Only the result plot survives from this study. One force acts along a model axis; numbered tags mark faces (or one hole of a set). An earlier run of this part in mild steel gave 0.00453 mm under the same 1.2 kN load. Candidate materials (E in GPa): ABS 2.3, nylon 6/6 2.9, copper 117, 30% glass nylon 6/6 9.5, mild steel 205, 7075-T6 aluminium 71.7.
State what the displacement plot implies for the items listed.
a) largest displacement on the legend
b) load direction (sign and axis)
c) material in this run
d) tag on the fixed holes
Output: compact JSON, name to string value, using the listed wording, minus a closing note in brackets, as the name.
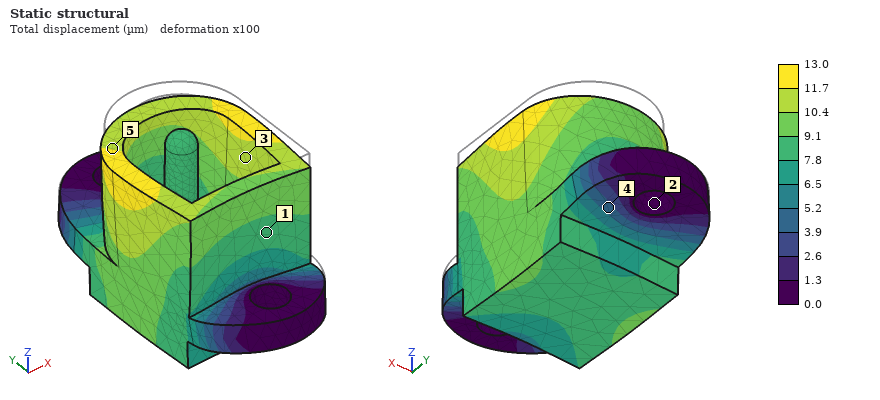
{"largest displacement on the legend": "13.0 µm", "load direction": "-Z", "material in this run": "7075-T6 aluminium", "tag on the fixed holes": "2"}
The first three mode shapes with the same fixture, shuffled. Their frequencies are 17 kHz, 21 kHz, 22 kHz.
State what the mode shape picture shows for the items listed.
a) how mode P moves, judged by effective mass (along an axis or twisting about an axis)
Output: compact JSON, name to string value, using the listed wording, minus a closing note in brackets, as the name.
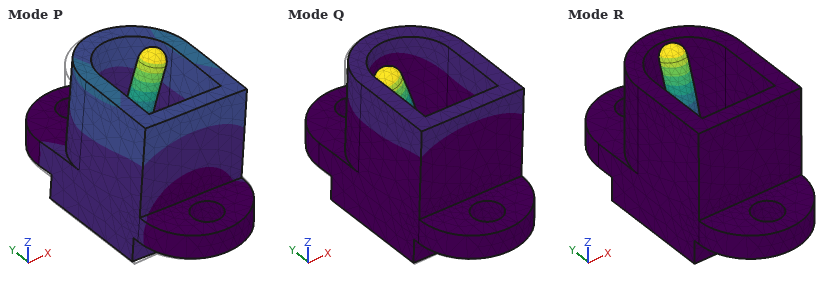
{"how mode P moves, judged by effective mass": "along X"}
